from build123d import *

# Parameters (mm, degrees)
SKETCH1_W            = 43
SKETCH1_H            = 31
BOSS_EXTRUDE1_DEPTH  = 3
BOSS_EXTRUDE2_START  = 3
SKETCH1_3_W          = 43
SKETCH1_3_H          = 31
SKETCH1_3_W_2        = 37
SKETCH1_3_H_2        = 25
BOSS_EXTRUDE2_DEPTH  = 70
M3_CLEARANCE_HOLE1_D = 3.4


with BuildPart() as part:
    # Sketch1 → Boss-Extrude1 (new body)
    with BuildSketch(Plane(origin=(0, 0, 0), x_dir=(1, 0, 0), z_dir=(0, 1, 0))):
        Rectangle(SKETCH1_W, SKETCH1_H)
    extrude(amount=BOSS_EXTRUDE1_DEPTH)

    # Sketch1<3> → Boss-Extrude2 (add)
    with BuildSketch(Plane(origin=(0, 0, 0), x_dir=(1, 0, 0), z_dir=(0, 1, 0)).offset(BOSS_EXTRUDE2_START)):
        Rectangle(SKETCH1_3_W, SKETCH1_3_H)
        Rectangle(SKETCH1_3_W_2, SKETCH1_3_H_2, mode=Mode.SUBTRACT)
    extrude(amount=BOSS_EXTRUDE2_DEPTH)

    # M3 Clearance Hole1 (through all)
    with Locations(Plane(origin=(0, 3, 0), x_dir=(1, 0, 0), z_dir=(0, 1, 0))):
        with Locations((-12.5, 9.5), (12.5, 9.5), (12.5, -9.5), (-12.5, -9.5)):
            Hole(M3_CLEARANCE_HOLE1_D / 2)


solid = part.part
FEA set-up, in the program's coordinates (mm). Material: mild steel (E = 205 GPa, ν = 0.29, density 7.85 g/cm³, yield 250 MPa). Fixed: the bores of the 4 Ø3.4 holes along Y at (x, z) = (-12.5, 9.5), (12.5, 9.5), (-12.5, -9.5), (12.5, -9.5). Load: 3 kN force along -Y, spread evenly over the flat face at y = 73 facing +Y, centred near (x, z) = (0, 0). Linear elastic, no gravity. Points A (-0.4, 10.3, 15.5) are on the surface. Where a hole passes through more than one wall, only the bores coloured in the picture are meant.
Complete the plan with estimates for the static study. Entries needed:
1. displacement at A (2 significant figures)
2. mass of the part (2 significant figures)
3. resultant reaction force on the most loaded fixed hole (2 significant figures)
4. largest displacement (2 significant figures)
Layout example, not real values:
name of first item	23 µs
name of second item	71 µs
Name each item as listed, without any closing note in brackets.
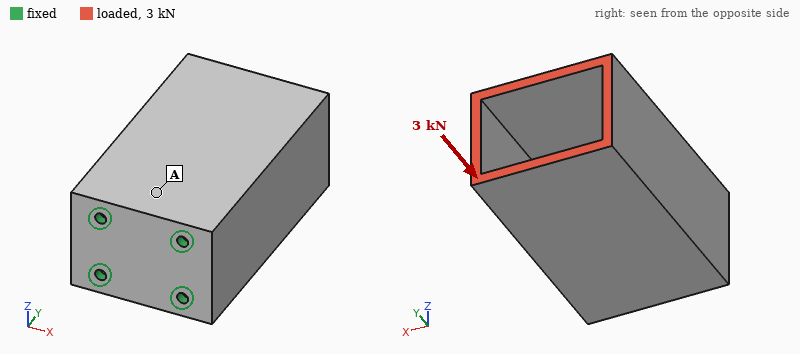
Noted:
displacement at A	2.9 µm
mass of the part	250 g
resultant reaction force on the most loaded fixed hole	750 N
largest displacement	4.7 µm
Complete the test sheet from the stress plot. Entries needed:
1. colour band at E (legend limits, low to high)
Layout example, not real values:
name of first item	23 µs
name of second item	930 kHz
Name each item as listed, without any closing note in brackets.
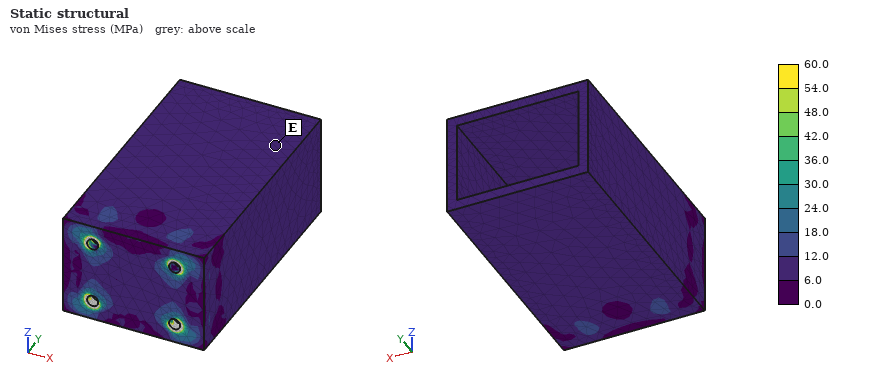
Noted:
colour band at E	6.0 to 12.0 MPa
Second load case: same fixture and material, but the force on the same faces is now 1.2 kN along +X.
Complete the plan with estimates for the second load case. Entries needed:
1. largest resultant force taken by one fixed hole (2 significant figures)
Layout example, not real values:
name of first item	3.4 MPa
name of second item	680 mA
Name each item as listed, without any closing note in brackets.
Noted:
largest resultant force taken by one fixed hole	1.6 kN
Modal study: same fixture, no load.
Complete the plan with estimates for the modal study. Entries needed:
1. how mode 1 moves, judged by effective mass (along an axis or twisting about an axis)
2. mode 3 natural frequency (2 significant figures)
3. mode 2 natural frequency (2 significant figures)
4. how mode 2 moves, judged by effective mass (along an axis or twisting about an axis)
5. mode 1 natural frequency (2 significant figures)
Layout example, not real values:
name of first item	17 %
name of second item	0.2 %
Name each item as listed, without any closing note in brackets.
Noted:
how mode 1 moves, judged by effective mass	along Z
mode 3 natural frequency	4200 Hz
mode 2 natural frequency	3100 Hz
how mode 2 moves, judged by effective mass	along X
mode 1 natural frequency	2600 Hz
